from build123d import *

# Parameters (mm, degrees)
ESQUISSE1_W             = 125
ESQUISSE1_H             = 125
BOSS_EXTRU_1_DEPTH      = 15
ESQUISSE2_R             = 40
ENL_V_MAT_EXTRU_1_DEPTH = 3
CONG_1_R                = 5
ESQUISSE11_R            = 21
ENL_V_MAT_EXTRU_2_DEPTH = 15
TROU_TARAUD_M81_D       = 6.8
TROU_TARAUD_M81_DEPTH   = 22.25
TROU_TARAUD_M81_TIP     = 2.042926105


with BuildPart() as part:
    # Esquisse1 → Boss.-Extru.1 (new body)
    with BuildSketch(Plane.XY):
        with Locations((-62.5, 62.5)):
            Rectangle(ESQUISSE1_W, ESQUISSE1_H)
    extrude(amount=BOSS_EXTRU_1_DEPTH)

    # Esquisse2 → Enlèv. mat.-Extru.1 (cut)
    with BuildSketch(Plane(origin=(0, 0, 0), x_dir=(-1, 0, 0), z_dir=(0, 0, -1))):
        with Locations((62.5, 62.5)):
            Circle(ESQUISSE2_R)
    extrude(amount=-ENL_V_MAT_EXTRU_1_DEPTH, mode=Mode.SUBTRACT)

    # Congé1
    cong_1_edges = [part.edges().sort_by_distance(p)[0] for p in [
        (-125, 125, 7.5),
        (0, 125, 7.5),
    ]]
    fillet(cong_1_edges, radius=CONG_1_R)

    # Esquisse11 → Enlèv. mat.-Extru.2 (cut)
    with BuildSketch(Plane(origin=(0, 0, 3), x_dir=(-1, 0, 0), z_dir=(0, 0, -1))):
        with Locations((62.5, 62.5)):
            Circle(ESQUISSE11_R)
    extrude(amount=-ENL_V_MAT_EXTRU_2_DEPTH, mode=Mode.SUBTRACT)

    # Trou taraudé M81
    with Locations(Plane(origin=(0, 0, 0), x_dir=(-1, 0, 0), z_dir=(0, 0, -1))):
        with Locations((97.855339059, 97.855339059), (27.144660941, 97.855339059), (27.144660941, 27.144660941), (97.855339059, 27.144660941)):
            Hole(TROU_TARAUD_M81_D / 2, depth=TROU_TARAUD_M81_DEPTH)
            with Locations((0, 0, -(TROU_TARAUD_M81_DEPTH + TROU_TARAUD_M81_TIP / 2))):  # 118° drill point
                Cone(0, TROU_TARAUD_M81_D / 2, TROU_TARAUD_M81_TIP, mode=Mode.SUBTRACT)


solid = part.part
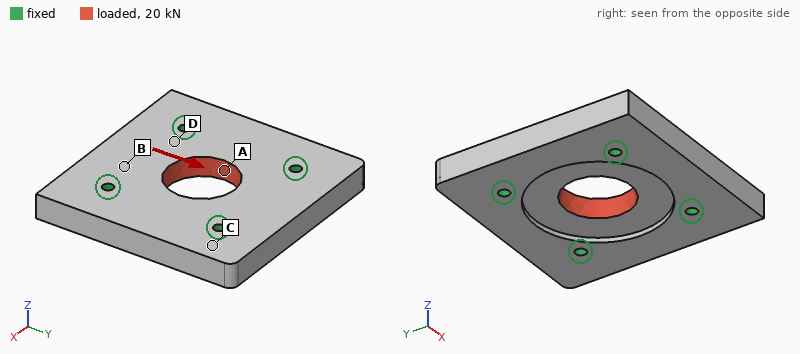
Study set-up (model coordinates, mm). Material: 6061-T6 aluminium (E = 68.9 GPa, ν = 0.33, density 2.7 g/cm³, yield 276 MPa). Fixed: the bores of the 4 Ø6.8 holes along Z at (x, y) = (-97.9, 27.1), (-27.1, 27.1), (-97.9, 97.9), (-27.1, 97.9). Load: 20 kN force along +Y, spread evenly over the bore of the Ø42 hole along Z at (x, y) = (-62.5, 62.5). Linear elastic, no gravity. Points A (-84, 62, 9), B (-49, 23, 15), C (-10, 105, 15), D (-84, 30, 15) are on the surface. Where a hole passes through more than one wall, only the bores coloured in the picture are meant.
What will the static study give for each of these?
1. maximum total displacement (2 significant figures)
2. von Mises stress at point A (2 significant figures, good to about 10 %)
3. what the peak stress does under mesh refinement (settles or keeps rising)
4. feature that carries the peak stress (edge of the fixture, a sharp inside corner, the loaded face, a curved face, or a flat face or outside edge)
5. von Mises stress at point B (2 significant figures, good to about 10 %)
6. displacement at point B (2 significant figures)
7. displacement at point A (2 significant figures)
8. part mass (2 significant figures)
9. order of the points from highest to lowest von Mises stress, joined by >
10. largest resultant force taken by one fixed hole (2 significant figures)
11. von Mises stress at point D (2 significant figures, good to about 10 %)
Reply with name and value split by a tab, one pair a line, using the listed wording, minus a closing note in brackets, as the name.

maximum total displacement	11 µm
von Mises stress at point A	22 MPa
what the peak stress does under mesh refinement	keeps rising
feature that carries the peak stress	edge of the fixture
von Mises stress at point B	8.6 MPa
displacement at point B	6.5 µm
displacement at point A	7.2 µm
part mass	540 g
order of the points from highest to lowest von Mises stress, joined by >	A > D > B > C
largest resultant force taken by one fixed hole	5.1 kN
von Mises stress at point D	11 MPa
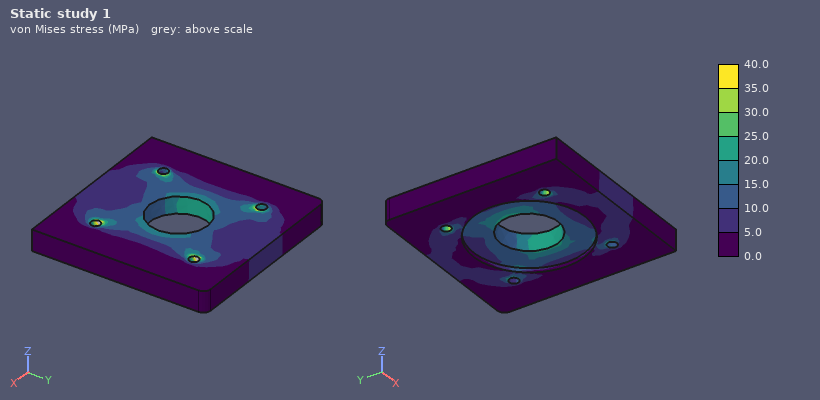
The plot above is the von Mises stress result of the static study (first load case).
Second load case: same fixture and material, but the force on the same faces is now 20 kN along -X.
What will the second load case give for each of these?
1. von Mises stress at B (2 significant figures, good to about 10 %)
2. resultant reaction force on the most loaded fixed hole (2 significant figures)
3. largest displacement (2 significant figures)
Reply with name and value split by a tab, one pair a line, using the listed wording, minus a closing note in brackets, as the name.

von Mises stress at B	4.9 MPa
resultant reaction force on the most loaded fixed hole	5.1 kN
largest displacement	11 µm
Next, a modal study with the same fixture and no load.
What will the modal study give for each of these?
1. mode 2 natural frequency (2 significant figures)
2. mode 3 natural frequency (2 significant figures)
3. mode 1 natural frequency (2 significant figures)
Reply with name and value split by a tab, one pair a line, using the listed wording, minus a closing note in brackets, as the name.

mode 2 natural frequency	9000 Hz
mode 3 natural frequency	9000 Hz
mode 1 natural frequency	7900 Hz
